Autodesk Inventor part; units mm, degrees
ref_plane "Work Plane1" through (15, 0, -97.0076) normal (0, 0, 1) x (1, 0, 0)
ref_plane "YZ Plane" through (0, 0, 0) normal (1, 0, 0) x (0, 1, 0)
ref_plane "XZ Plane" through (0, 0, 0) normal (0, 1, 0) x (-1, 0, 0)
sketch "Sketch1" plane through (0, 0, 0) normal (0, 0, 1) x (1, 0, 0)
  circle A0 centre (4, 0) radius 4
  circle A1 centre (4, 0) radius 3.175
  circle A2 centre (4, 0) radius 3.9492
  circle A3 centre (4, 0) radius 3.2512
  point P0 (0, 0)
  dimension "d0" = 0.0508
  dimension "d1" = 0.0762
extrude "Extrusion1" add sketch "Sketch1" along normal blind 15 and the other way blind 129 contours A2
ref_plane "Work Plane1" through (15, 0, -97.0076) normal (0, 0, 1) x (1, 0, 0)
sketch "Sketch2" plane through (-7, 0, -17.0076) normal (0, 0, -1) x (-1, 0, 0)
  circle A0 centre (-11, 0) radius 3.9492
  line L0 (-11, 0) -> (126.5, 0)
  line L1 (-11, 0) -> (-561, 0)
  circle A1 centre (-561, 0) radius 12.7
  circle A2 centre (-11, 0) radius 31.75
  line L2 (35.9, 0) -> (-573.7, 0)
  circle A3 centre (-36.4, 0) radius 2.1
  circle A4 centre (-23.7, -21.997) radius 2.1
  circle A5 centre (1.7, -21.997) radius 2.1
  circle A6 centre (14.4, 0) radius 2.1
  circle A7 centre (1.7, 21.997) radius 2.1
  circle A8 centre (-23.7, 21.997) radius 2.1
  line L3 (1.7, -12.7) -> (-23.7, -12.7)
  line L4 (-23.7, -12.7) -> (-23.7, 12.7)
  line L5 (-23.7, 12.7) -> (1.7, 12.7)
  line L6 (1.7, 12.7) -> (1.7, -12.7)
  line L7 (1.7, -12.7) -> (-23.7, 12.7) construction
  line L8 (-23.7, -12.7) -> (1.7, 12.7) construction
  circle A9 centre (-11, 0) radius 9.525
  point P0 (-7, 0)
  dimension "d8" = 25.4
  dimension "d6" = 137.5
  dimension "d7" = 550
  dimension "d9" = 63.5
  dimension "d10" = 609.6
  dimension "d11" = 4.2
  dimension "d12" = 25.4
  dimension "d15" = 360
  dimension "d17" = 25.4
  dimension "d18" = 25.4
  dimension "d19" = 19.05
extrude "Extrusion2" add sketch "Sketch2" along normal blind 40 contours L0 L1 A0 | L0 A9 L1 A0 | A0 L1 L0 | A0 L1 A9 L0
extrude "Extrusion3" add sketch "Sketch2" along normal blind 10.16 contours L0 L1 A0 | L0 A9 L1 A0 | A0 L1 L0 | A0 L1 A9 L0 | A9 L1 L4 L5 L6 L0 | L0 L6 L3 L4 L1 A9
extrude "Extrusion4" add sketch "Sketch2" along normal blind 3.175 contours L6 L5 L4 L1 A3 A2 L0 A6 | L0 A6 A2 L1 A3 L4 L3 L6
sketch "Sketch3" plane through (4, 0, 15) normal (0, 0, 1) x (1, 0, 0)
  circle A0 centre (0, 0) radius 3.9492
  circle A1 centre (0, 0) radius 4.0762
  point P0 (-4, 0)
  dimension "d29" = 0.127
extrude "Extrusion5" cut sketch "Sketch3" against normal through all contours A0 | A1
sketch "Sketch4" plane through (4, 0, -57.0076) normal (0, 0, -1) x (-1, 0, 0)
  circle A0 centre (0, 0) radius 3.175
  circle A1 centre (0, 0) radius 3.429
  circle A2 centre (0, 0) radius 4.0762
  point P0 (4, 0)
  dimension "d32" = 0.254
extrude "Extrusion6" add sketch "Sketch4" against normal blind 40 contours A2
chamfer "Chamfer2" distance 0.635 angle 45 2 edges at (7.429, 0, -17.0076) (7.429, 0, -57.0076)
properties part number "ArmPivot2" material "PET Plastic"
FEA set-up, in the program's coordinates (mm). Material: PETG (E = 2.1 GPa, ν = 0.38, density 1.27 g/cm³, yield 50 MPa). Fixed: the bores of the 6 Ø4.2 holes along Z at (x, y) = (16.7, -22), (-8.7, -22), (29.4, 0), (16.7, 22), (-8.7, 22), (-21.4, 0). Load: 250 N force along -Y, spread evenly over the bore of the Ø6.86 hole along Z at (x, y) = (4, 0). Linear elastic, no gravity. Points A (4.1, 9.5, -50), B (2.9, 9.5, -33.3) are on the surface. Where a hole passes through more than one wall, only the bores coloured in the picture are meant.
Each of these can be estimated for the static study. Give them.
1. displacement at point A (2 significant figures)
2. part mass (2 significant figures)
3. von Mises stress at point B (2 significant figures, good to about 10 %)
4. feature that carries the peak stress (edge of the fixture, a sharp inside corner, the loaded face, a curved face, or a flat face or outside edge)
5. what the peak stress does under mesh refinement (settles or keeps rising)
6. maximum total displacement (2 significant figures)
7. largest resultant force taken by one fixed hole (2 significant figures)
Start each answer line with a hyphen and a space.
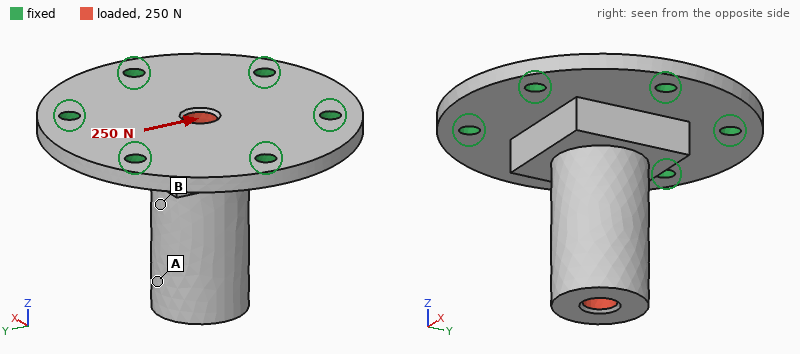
- 0.28 mm
- 27 g
- 2.5 MPa
- edge of the fixture
- keeps rising
- 0.34 mm
- 88 N
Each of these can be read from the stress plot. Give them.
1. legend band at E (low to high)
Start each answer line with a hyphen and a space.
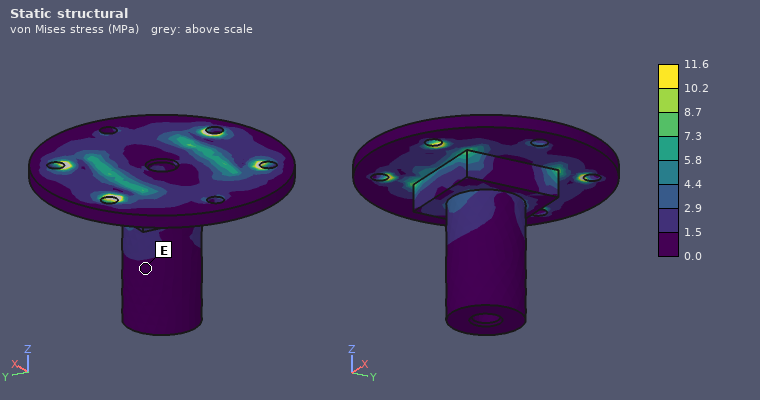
- 0.0 to 1.5 MPa
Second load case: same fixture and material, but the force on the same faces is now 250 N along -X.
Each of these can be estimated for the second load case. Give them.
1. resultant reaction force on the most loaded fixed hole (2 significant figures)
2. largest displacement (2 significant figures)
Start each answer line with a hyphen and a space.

- 86 N
- 0.35 mm
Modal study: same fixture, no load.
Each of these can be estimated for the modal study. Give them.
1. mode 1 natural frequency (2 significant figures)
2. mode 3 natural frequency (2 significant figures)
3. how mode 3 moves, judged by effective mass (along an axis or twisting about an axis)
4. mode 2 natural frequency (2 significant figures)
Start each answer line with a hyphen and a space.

- 1400 Hz
- 2100 Hz
- along Z
- 1400 Hz
